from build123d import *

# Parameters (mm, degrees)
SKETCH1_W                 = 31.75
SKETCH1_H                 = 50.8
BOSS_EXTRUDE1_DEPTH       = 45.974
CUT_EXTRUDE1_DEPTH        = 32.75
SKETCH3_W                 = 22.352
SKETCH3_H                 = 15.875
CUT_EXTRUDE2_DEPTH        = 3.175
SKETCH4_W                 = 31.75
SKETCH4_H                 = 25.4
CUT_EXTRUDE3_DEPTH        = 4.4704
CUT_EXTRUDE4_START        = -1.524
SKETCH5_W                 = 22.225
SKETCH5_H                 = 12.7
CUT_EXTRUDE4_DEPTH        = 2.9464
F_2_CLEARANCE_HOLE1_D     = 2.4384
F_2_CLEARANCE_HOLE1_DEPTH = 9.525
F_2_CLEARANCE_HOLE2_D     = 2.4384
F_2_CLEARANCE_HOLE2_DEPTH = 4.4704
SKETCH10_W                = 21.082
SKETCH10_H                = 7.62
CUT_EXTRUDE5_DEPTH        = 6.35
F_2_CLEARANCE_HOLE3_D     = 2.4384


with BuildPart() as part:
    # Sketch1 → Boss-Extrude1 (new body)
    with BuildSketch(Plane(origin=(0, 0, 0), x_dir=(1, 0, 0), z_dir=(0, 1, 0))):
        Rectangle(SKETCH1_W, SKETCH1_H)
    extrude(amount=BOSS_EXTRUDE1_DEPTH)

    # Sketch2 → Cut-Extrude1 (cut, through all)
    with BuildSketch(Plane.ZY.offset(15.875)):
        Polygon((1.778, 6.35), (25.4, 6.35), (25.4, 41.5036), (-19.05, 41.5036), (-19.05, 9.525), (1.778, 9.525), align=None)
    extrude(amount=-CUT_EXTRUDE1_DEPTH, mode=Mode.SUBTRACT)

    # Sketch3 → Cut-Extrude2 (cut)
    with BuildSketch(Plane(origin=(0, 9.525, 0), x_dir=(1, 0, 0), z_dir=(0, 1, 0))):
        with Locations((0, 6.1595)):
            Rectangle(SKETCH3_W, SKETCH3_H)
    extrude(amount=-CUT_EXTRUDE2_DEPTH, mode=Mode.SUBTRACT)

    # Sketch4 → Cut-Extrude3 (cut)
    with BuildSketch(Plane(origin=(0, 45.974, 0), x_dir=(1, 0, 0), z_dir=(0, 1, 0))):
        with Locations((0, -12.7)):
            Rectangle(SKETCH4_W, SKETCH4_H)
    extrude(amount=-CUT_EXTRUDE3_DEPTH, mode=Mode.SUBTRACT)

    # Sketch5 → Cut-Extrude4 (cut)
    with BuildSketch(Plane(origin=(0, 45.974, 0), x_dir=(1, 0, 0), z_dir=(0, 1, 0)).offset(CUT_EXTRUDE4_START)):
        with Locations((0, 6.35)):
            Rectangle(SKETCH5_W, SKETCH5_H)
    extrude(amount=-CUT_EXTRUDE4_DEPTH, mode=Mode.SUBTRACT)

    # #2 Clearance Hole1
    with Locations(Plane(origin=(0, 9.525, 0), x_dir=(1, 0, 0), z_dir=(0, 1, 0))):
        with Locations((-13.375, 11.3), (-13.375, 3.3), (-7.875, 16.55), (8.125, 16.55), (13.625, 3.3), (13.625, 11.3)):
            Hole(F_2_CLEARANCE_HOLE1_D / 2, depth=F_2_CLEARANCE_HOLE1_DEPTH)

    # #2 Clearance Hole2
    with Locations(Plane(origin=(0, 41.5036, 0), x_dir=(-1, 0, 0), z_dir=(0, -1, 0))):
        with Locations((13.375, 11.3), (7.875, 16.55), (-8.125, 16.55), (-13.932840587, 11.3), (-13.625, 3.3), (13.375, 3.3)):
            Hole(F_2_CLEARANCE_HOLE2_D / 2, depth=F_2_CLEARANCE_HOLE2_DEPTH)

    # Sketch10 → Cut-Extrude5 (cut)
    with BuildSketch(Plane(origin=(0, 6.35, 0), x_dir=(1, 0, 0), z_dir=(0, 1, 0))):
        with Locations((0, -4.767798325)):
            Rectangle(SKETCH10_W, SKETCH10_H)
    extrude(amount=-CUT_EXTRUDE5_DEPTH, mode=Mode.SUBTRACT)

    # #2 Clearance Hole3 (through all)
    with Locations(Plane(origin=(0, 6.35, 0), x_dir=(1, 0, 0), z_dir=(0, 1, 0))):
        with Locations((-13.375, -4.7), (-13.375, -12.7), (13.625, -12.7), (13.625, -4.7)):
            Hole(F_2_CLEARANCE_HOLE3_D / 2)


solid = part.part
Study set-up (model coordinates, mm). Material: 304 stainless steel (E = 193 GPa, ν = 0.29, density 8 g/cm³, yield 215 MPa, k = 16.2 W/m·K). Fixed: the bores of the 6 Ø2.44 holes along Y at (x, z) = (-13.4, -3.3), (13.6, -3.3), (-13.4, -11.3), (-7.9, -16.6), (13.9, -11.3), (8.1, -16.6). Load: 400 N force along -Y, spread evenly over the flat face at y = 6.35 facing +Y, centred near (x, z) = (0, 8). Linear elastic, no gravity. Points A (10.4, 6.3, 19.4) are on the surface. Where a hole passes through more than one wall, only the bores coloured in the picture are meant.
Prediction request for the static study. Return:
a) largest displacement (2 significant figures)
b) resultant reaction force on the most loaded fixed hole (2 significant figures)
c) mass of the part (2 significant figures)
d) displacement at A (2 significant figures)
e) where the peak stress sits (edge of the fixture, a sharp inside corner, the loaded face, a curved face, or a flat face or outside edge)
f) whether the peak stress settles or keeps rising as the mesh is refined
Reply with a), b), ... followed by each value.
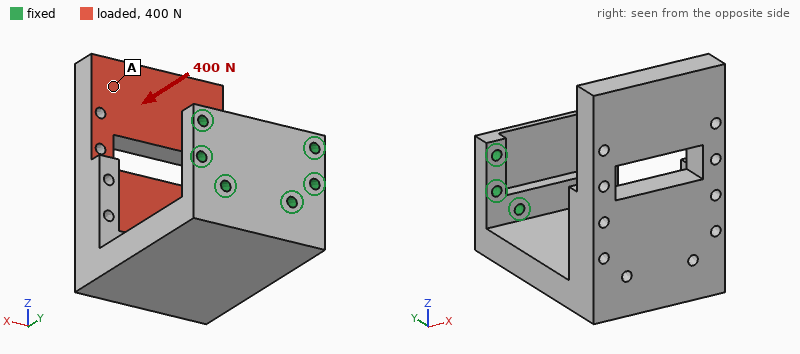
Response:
a) 0.29 mm
b) 210 N
c) 160 g
d) 0.24 mm
e) edge of the fixture
f) keeps rising
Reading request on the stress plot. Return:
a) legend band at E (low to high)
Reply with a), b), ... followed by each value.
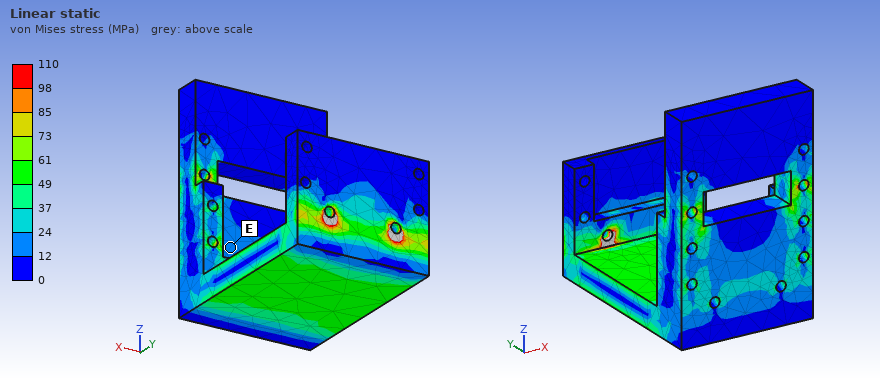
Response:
a) 12 to 24 MPa
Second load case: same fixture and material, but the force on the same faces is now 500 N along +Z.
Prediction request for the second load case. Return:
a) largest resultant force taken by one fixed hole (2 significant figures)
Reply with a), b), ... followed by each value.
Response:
a) 490 N
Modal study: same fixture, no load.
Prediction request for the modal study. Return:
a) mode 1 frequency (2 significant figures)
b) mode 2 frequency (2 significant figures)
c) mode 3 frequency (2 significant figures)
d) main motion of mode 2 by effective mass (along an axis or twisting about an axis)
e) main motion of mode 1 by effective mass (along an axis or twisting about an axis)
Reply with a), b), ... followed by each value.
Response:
a) 720 Hz
b) 1300 Hz
c) 2200 Hz
d) along X
e) along Z
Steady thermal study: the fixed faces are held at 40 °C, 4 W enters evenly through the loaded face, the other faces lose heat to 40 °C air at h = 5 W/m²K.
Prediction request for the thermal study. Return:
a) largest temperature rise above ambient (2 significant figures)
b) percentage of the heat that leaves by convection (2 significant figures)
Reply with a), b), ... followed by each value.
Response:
a) 83 K
b) 35 %
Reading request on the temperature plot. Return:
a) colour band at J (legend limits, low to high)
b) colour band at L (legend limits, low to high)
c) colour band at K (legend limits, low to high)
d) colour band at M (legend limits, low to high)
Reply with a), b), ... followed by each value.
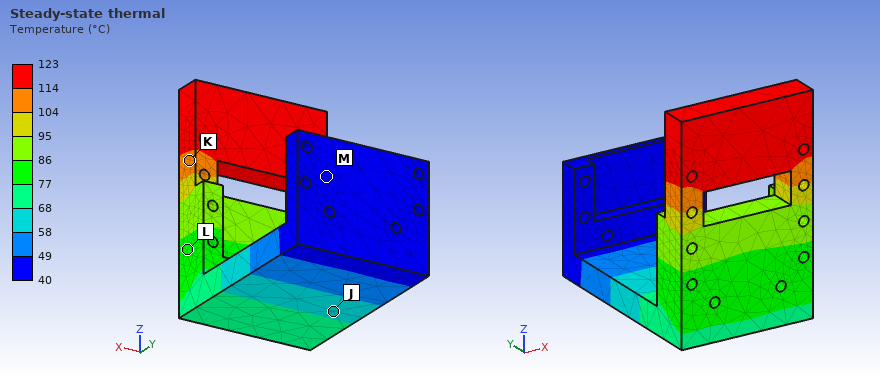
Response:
a) 58 to 68 °C
b) 77 to 86 °C
c) 104 to 114 °C
d) 40 to 49 °C
